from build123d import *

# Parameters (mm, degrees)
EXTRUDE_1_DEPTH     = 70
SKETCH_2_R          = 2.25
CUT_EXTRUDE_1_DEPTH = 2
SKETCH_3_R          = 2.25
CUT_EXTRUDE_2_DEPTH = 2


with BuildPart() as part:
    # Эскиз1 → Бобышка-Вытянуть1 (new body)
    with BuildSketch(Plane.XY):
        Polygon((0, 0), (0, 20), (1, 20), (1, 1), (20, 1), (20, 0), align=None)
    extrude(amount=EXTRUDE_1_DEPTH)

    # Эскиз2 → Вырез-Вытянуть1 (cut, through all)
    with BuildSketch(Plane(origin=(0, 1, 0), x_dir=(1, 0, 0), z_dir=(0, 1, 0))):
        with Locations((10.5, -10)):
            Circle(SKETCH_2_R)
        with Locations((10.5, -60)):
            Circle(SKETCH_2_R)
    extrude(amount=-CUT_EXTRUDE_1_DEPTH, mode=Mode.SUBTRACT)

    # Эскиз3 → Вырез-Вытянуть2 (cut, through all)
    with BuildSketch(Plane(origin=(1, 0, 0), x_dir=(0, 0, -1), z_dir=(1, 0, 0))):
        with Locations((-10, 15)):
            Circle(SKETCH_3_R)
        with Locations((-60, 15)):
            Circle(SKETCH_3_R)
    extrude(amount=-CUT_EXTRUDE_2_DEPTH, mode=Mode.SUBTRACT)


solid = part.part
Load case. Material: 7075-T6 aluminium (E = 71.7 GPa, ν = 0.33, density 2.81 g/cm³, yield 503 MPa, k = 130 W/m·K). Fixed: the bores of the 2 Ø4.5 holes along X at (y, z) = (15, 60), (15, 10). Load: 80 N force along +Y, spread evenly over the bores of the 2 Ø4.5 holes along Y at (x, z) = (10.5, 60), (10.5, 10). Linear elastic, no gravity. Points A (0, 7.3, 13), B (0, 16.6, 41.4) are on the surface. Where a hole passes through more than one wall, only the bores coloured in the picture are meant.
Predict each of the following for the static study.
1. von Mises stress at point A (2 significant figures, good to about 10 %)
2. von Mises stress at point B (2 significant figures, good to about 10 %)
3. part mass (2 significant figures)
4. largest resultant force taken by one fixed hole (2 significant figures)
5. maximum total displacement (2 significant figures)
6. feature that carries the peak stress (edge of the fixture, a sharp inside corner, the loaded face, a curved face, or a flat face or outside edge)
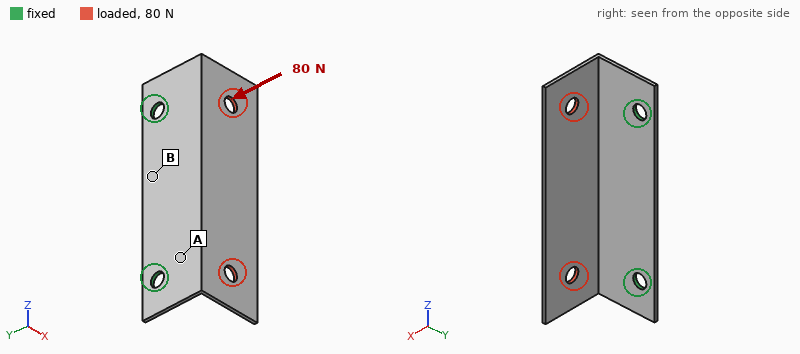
76 MPa
24 MPa
7.5 g
40 N
0.82 mm
a flat face or outside edge
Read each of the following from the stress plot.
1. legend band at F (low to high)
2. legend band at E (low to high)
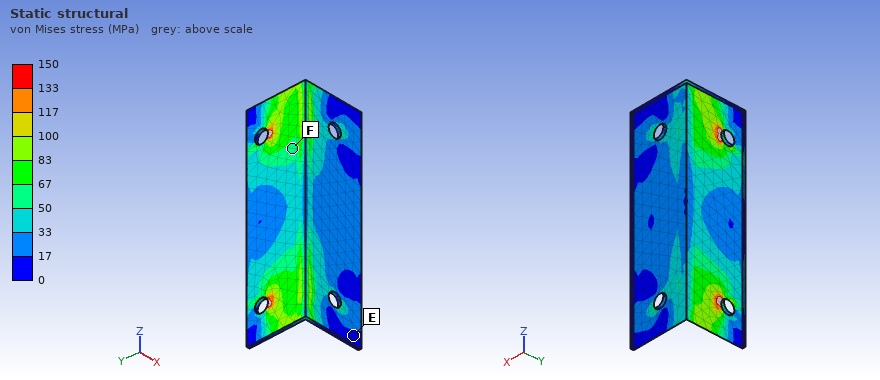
50 to 67 MPa
0 to 17 MPa
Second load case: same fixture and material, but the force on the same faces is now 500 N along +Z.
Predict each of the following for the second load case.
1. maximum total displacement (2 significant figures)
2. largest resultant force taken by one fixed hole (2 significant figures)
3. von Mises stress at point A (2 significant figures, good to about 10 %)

0.89 mm
300 N
120 MPa
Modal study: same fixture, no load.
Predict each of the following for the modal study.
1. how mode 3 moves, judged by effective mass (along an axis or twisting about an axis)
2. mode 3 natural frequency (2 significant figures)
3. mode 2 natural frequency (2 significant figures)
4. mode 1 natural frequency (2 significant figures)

along X
2200 Hz
1400 Hz
900 Hz
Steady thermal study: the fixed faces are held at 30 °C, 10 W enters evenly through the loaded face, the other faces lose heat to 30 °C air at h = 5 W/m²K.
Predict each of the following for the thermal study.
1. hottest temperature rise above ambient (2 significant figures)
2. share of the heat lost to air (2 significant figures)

43 K
6.0 %
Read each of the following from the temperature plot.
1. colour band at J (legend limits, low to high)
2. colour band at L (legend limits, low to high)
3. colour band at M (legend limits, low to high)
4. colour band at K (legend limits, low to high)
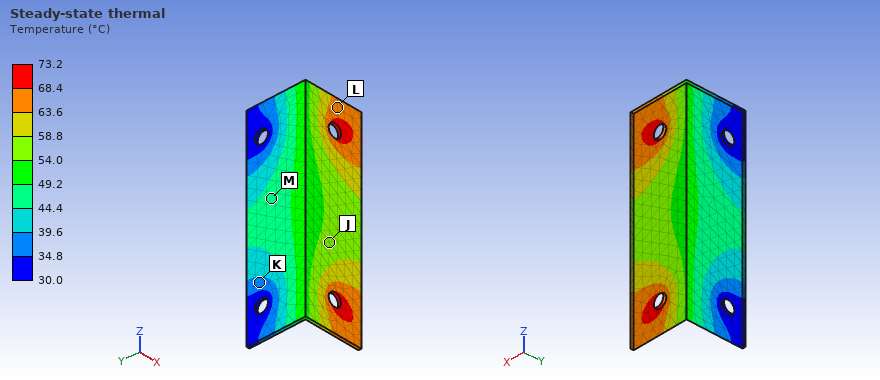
54.0 to 58.8 °C
63.6 to 68.4 °C
44.4 to 49.2 °C
34.8 to 39.6 °C
